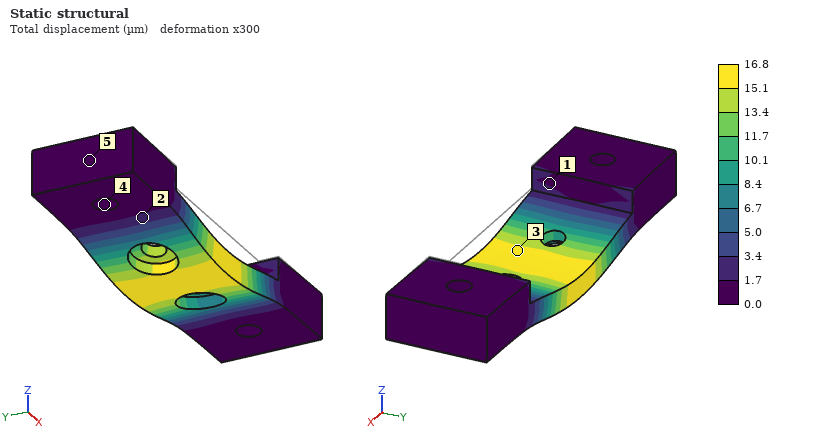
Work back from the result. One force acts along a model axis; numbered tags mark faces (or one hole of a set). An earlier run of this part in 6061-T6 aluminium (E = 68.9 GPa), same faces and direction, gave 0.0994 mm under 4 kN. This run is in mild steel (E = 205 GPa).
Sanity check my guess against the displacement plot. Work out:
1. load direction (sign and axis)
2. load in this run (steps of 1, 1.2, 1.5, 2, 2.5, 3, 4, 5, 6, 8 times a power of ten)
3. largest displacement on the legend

-Z
2 kN
16.8 µm
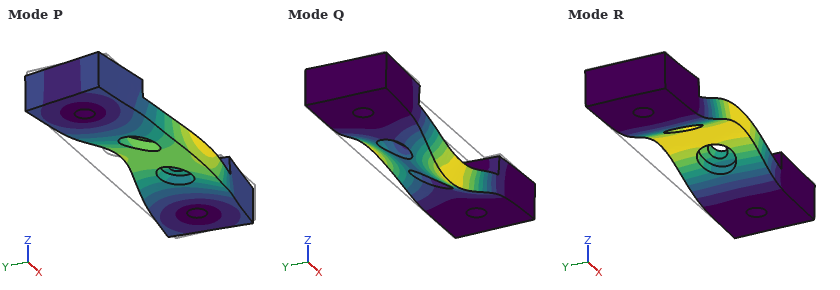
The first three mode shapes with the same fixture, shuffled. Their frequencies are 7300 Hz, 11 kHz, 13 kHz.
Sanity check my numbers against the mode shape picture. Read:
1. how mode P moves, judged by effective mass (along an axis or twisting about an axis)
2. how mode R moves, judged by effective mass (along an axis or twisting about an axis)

along Y
along Z
